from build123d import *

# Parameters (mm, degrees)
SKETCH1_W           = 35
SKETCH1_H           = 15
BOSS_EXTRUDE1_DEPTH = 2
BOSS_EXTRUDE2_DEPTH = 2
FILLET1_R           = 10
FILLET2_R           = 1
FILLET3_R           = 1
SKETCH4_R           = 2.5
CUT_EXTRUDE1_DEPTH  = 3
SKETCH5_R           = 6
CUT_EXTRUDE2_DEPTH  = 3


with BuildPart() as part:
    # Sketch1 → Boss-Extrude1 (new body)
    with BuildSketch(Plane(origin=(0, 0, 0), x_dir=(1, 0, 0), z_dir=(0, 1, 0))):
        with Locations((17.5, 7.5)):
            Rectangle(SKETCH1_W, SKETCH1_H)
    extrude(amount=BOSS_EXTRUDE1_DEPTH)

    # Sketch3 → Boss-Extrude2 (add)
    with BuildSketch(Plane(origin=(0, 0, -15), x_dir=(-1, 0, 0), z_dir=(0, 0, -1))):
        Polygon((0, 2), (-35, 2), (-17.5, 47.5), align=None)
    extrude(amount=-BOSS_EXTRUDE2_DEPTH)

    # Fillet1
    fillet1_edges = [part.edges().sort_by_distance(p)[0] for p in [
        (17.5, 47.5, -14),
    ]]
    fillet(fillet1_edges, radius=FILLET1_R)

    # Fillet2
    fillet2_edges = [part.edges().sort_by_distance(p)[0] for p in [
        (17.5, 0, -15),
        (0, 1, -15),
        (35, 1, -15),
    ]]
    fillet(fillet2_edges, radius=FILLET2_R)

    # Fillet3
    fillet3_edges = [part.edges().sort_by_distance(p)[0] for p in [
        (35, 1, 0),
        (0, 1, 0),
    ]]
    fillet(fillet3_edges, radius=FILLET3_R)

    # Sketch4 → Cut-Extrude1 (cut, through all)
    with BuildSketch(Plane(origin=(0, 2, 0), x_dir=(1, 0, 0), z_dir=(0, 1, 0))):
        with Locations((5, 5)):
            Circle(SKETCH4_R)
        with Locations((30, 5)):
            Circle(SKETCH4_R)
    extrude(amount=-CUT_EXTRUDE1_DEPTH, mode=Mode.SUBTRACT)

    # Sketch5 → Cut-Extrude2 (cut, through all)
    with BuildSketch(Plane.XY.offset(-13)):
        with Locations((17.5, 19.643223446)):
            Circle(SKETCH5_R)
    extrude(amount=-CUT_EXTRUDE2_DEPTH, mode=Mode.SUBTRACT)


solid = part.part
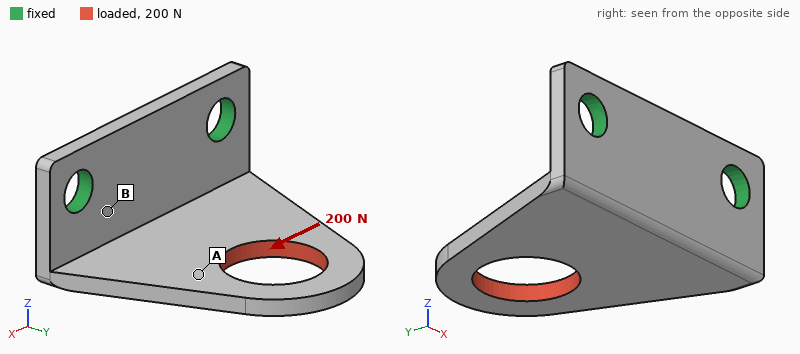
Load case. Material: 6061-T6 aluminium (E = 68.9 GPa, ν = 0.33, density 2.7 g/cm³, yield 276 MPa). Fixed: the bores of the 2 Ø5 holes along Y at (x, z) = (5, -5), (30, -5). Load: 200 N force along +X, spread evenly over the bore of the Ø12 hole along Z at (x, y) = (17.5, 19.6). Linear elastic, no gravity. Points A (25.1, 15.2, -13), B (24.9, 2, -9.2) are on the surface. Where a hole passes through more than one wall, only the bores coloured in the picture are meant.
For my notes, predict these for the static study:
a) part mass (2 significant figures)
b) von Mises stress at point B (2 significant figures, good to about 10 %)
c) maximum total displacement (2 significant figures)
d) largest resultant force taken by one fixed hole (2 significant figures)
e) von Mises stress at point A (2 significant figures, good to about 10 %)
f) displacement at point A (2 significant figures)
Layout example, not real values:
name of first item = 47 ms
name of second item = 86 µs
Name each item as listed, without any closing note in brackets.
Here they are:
part mass = 5.5 g
von Mises stress at point B = 32 MPa
maximum total displacement = 61 µm
largest resultant force taken by one fixed hole = 180 N
von Mises stress at point A = 9.8 MPa
displacement at point A = 36 µm
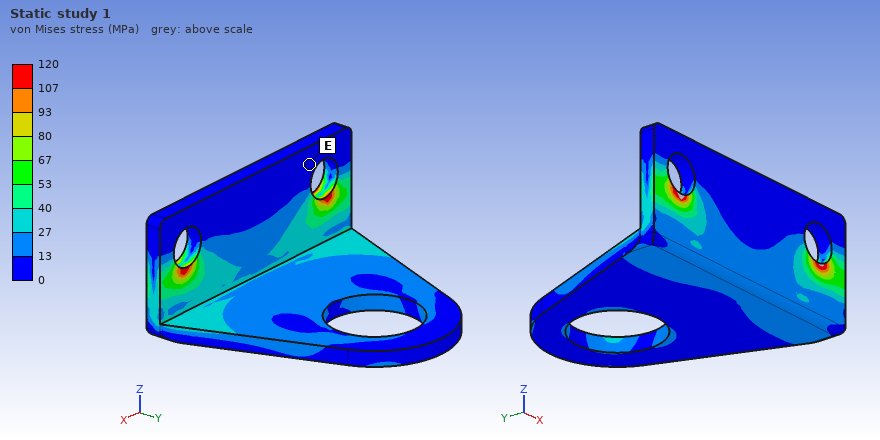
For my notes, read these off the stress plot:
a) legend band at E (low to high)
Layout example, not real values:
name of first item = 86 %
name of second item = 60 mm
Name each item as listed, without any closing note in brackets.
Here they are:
legend band at E = 0 to 13 MPa
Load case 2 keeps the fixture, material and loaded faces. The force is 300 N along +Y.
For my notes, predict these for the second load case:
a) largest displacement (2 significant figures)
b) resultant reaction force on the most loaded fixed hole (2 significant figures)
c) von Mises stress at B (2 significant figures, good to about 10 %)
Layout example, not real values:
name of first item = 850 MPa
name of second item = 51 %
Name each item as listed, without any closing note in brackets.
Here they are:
largest displacement = 0.16 mm
resultant reaction force on the most loaded fixed hole = 150 N
von Mises stress at B = 45 MPa
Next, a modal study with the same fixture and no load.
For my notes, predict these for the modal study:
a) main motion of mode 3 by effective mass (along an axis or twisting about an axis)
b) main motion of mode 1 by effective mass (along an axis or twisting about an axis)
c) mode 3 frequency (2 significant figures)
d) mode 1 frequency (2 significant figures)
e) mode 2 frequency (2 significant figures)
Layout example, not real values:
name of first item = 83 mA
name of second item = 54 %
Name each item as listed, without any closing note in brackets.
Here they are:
main motion of mode 3 by effective mass = along Y
main motion of mode 1 by effective mass = along Z
mode 3 frequency = 8100 Hz
mode 1 frequency = 2300 Hz
mode 2 frequency = 6300 Hz
